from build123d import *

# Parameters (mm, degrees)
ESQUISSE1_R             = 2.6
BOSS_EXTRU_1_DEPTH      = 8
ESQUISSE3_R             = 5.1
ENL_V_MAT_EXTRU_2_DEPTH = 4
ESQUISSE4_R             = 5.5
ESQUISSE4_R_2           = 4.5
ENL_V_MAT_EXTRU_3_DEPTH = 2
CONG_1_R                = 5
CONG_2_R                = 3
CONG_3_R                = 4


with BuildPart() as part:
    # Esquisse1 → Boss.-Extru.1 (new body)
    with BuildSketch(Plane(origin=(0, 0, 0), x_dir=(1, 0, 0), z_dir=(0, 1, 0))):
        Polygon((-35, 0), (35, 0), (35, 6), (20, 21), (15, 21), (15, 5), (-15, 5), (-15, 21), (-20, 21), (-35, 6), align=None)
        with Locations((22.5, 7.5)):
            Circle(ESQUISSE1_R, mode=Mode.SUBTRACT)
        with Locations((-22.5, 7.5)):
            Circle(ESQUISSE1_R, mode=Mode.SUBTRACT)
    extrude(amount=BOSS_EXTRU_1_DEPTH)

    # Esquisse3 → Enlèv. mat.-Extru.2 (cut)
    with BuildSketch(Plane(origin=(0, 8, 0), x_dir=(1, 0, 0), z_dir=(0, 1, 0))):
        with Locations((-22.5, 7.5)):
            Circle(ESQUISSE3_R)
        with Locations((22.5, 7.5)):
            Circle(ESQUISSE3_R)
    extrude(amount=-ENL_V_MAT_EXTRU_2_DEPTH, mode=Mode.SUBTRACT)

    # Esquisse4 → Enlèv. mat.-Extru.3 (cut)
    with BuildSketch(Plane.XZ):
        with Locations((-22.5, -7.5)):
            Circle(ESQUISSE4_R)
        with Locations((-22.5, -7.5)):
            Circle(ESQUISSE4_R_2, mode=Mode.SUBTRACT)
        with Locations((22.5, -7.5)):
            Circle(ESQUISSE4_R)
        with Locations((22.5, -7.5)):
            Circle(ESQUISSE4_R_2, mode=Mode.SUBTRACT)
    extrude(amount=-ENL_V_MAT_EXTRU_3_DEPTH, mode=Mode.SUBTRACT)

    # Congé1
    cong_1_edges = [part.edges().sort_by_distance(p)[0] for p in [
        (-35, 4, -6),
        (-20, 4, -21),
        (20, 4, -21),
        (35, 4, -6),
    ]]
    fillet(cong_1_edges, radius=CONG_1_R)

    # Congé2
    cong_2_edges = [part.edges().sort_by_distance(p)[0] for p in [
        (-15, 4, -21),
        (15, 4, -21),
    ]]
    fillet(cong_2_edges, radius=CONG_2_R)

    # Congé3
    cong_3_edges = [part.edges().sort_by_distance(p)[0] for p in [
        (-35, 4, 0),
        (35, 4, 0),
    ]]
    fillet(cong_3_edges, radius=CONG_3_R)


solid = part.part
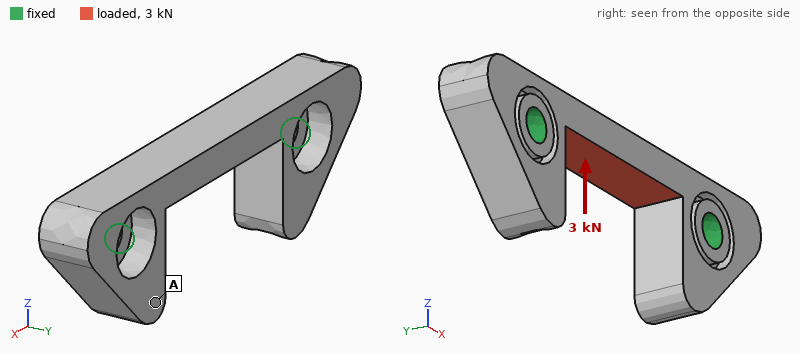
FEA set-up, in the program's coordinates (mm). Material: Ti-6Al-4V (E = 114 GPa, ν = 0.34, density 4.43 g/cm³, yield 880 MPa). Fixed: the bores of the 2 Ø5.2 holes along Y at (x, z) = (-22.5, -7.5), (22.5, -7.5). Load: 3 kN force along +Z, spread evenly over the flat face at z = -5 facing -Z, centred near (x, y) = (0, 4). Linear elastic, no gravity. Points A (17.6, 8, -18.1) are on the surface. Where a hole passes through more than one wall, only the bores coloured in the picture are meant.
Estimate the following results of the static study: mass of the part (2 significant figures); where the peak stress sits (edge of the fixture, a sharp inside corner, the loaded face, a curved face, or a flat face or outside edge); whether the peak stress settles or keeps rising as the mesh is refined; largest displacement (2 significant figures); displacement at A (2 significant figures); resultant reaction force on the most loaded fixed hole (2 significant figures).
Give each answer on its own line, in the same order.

22 g
edge of the fixture
keeps rising
73 µm
15 µm
1.8 kN
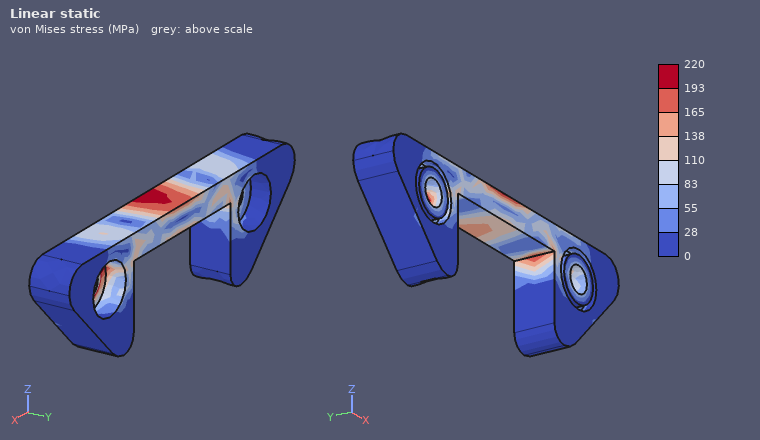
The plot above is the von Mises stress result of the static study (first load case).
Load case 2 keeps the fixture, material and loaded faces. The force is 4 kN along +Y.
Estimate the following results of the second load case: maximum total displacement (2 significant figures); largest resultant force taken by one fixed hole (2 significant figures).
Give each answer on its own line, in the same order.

0.11 mm
2.1 kN
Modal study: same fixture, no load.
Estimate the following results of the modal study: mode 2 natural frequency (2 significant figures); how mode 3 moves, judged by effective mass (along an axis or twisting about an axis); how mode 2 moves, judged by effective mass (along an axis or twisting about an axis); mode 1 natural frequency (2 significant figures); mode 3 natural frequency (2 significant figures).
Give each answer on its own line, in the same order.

16 kHz
twisting about X
along Z
13 kHz
17 kHz
